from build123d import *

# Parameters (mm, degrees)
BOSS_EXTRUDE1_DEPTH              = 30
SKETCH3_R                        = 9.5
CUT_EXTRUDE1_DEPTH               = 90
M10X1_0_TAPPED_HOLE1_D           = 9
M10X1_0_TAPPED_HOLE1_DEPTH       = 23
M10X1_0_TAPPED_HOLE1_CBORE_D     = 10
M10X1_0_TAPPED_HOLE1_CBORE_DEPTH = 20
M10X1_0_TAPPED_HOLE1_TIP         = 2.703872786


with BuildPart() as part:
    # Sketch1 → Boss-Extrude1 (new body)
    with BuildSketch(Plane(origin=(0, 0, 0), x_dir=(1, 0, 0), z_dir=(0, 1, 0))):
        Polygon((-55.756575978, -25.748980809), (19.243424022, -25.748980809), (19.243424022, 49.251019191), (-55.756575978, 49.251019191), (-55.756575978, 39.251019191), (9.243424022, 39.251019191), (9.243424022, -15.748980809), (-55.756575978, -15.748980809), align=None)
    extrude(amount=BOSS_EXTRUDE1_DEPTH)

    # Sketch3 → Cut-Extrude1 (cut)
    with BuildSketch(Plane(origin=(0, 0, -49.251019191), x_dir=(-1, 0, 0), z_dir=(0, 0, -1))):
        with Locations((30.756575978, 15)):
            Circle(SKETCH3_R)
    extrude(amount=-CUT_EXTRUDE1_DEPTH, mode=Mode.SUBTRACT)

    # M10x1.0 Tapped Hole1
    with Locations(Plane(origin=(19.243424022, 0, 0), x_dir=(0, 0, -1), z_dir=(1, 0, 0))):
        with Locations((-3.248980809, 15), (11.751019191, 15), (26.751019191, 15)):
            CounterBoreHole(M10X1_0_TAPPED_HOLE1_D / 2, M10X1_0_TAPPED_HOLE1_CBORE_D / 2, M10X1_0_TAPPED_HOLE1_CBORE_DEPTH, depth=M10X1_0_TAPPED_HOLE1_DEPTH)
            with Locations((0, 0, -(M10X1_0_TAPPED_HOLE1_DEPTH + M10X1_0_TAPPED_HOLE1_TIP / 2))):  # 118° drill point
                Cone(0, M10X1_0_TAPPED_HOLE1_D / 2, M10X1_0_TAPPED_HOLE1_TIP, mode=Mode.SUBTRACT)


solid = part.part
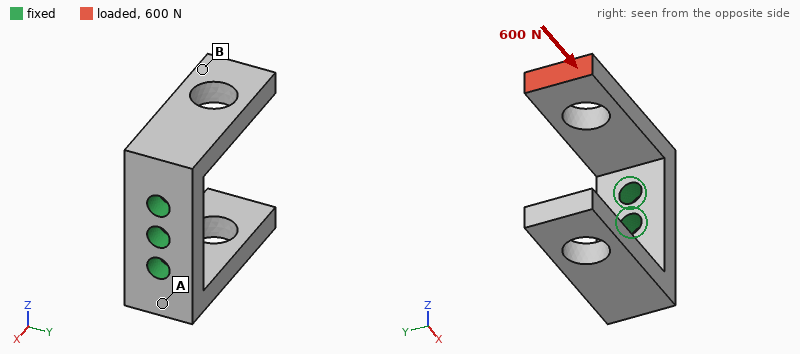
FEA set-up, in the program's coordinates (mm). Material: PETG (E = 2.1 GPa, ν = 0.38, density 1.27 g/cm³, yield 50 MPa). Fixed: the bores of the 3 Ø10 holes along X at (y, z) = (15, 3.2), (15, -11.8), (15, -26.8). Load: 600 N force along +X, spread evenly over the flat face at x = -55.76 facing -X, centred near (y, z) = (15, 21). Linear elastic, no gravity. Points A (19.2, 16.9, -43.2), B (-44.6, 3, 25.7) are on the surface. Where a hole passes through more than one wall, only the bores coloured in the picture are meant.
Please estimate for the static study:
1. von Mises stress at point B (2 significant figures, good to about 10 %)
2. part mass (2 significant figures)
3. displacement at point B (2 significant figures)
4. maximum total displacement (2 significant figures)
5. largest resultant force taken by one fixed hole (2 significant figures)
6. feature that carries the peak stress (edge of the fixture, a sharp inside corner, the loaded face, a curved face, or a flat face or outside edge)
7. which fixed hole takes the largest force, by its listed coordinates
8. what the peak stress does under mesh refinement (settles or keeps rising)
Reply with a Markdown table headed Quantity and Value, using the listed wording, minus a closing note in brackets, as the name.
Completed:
| Quantity | Value |
|---|---|
| von Mises stress at point B | 3.6 MPa |
| part mass | 68 g |
| displacement at point B | 0.90 mm |
| maximum total displacement | 1.1 mm |
| largest resultant force taken by one fixed hole | 690 N |
| feature that carries the peak stress | edge of the fixture |
| which fixed hole takes the largest force, by its listed coordinates | (15, 3.2) |
| what the peak stress does under mesh refinement | keeps rising |
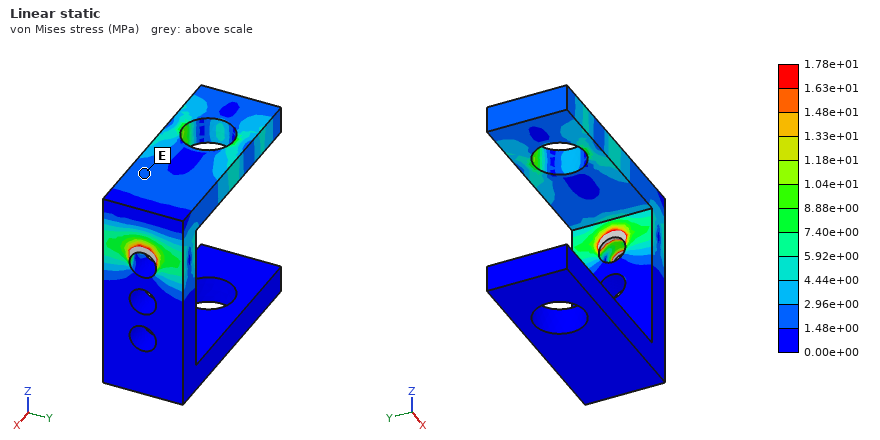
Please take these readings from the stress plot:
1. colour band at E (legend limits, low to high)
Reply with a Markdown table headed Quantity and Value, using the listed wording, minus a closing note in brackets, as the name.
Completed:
| Quantity | Value |
|---|---|
| colour band at E | 1.48e+00 to 2.96e+00 MPa |
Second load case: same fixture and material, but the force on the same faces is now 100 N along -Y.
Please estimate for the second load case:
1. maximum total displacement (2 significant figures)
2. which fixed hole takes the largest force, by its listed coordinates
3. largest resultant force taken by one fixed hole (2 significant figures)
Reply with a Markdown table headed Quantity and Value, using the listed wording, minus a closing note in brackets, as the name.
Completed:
| Quantity | Value |
|---|---|
| maximum total displacement | 1.2 mm |
| which fixed hole takes the largest force, by its listed coordinates | (15, 3.2) |
| largest resultant force taken by one fixed hole | 130 N |
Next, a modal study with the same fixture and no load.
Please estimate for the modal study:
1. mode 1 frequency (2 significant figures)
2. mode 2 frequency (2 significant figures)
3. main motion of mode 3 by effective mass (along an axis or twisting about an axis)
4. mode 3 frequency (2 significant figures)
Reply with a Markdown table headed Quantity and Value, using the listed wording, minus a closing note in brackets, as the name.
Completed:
| Quantity | Value |
|---|---|
| mode 1 frequency | 350 Hz |
| mode 2 frequency | 350 Hz |
| main motion of mode 3 by effective mass | twisting about X |
| mode 3 frequency | 550 Hz |
